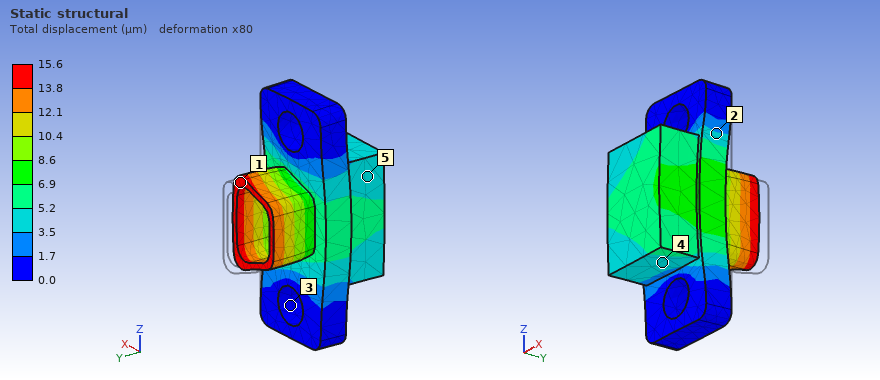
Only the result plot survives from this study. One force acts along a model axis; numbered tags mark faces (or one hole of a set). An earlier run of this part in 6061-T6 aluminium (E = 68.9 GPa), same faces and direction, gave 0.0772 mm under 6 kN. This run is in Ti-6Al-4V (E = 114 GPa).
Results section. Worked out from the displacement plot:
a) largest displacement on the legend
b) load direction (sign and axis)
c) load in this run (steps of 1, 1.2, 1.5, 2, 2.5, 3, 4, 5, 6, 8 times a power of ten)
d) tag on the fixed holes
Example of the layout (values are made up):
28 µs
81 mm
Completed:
15.6 µm
-Y
2 kN
3
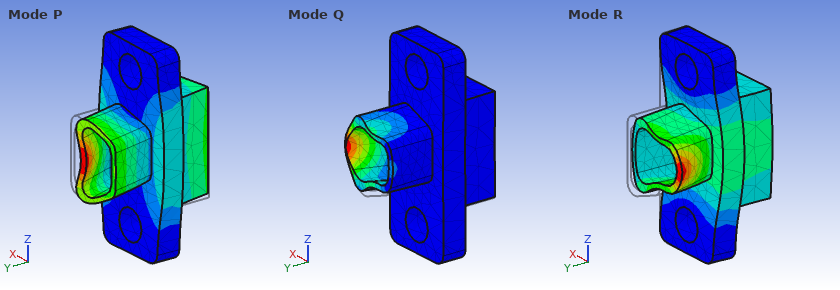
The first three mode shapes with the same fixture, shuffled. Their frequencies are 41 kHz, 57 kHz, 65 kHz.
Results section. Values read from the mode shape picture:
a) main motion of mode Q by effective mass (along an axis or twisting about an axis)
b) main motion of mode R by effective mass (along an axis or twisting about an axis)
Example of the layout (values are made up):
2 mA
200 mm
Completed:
along X
along Y
